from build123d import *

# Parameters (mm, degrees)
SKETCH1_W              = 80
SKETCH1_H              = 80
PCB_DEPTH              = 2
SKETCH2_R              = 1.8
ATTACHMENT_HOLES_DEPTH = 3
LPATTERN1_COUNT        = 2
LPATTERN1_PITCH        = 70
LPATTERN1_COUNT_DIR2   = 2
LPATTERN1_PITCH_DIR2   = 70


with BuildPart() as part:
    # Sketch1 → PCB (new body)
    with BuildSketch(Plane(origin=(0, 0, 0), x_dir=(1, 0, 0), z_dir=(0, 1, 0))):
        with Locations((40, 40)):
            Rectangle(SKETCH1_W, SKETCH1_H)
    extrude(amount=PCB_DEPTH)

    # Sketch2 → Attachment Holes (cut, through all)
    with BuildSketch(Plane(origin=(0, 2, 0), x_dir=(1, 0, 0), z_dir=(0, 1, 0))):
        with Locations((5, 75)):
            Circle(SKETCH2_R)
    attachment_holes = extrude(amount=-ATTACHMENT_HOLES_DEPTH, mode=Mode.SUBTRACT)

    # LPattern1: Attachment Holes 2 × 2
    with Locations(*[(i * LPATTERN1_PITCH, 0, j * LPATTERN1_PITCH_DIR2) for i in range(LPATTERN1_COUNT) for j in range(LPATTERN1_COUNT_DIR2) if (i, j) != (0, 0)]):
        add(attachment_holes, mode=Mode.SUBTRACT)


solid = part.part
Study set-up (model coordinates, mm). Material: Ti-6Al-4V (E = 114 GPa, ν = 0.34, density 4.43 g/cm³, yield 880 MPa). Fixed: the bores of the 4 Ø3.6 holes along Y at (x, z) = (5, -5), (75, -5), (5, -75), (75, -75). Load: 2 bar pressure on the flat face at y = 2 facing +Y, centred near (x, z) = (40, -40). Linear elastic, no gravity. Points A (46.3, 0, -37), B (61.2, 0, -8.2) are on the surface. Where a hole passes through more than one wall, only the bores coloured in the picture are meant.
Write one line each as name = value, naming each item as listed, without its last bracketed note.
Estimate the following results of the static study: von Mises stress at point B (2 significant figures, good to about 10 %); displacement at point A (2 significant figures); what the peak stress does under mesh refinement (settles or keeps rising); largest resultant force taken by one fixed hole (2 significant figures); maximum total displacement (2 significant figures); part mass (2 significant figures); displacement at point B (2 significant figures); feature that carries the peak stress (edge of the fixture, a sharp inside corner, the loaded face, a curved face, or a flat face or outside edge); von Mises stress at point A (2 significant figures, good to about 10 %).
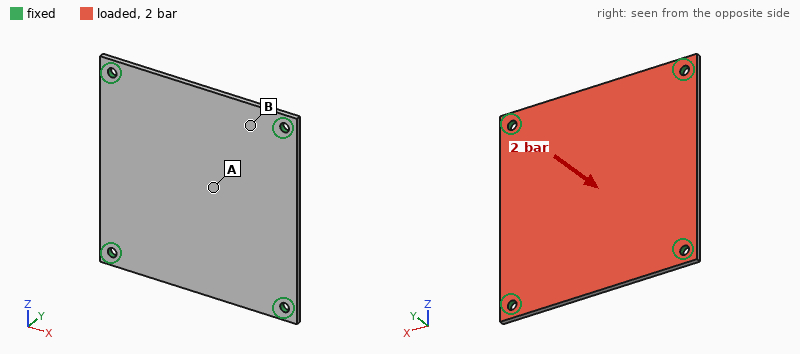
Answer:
von Mises stress at point B = 31 MPa
displacement at point A = 0.42 mm
what the peak stress does under mesh refinement = keeps rising
largest resultant force taken by one fixed hole = 320 N
maximum total displacement = 0.43 mm
part mass = 56 g
displacement at point B = 0.12 mm
feature that carries the peak stress = edge of the fixture
von Mises stress at point A = 81 MPa
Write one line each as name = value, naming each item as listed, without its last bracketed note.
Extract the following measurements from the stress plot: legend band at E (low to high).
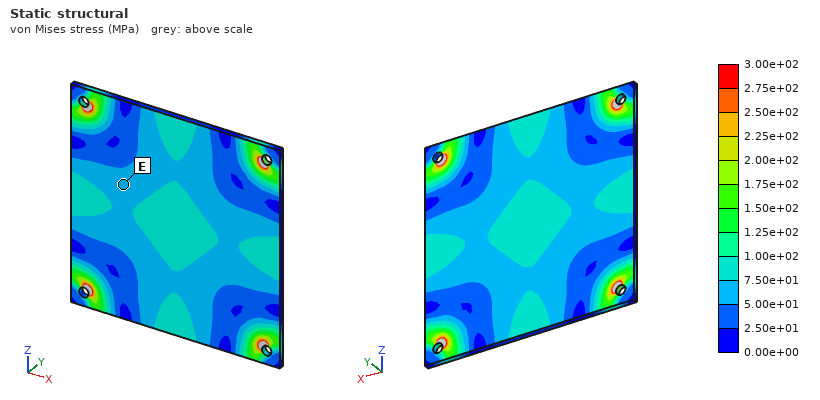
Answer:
legend band at E = 5.00e+01 to 7.50e+01 MPa
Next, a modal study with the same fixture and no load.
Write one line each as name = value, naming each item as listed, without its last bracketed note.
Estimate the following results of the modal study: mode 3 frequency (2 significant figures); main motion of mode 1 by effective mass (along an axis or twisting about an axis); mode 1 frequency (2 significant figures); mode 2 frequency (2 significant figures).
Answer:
mode 3 frequency = 2400 Hz
main motion of mode 1 by effective mass = along Y
mode 1 frequency = 1400 Hz
mode 2 frequency = 2400 Hz
